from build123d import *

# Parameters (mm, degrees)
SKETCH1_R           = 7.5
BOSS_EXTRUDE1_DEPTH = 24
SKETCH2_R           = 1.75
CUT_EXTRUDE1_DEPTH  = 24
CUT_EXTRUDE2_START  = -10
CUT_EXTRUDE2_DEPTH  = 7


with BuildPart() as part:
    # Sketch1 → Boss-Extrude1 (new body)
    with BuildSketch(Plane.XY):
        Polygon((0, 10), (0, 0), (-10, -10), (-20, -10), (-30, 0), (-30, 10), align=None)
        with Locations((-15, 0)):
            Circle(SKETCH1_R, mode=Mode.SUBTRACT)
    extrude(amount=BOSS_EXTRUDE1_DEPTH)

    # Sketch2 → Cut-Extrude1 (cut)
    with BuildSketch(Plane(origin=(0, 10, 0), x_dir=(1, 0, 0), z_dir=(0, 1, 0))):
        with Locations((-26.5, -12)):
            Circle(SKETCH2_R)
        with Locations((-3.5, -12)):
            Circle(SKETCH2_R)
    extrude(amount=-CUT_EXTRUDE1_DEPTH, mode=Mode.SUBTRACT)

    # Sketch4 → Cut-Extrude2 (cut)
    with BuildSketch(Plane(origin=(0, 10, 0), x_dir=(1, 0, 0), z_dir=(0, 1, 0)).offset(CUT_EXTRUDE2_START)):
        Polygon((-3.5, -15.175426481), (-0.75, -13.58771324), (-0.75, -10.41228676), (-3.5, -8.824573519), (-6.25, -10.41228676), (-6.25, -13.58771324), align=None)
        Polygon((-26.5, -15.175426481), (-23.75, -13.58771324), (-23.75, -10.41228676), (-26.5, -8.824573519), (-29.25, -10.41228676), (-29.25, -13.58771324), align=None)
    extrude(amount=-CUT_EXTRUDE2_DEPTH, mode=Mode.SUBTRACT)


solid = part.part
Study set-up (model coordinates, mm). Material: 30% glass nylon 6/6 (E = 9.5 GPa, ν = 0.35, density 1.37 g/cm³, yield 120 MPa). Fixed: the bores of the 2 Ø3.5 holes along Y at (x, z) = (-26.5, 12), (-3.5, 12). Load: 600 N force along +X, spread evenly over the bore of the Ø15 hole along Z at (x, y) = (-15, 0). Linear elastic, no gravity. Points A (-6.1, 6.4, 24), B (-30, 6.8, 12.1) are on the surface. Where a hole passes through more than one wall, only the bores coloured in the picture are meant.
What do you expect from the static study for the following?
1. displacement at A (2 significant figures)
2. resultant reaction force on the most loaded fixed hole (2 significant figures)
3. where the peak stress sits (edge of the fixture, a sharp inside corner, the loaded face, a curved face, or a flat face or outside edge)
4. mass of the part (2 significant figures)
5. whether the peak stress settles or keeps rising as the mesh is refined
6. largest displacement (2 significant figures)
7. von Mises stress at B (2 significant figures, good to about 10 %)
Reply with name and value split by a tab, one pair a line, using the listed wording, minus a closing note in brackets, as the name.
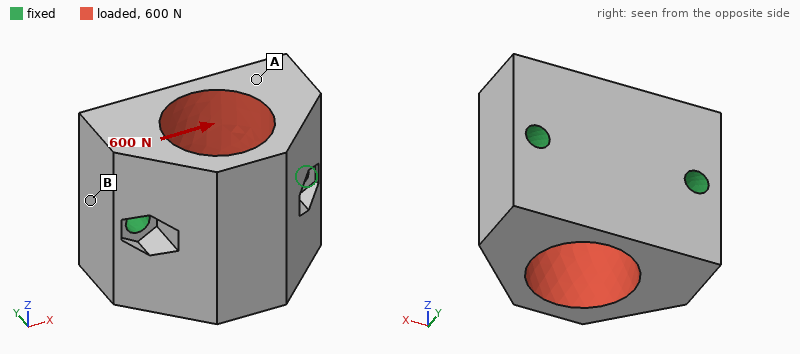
displacement at A	3.2 µm
resultant reaction force on the most loaded fixed hole	310 N
where the peak stress sits	edge of the fixture
mass of the part	10 g
whether the peak stress settles or keeps rising as the mesh is refined	keeps rising
largest displacement	14 µm
von Mises stress at B	3.1 MPa
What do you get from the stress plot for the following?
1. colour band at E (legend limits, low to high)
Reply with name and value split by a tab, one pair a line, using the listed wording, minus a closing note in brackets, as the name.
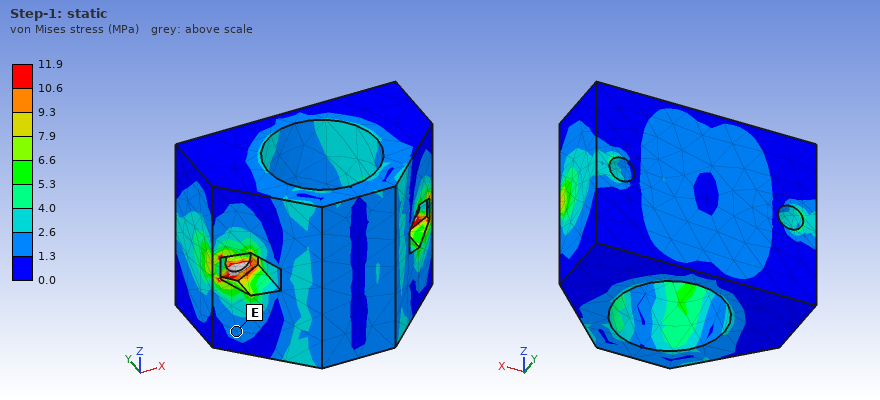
colour band at E	1.3 to 2.6 MPa
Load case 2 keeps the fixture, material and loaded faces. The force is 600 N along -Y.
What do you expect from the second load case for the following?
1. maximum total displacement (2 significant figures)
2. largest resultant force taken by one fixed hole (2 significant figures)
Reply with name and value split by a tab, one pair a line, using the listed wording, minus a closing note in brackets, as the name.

maximum total displacement	8.4 µm
largest resultant force taken by one fixed hole	300 N
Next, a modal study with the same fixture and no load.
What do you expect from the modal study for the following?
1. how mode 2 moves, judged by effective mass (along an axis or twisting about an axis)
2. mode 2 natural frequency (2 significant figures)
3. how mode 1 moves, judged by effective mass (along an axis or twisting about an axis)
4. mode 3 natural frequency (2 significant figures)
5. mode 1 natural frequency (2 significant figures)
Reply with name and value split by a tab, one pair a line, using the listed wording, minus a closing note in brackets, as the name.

how mode 2 moves, judged by effective mass	along X
mode 2 natural frequency	14 kHz
how mode 1 moves, judged by effective mass	along Z
mode 3 natural frequency	17 kHz
mode 1 natural frequency	11 kHz
